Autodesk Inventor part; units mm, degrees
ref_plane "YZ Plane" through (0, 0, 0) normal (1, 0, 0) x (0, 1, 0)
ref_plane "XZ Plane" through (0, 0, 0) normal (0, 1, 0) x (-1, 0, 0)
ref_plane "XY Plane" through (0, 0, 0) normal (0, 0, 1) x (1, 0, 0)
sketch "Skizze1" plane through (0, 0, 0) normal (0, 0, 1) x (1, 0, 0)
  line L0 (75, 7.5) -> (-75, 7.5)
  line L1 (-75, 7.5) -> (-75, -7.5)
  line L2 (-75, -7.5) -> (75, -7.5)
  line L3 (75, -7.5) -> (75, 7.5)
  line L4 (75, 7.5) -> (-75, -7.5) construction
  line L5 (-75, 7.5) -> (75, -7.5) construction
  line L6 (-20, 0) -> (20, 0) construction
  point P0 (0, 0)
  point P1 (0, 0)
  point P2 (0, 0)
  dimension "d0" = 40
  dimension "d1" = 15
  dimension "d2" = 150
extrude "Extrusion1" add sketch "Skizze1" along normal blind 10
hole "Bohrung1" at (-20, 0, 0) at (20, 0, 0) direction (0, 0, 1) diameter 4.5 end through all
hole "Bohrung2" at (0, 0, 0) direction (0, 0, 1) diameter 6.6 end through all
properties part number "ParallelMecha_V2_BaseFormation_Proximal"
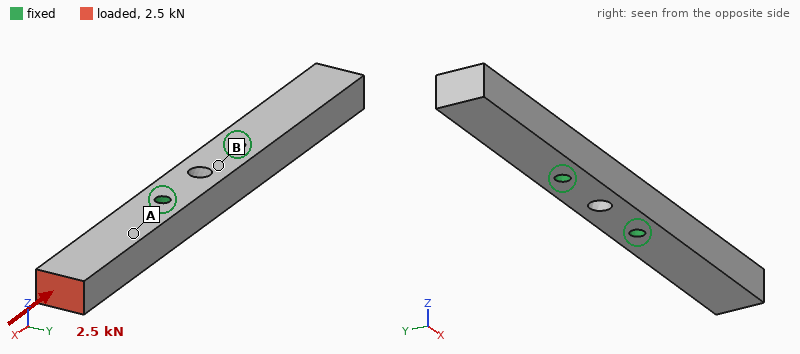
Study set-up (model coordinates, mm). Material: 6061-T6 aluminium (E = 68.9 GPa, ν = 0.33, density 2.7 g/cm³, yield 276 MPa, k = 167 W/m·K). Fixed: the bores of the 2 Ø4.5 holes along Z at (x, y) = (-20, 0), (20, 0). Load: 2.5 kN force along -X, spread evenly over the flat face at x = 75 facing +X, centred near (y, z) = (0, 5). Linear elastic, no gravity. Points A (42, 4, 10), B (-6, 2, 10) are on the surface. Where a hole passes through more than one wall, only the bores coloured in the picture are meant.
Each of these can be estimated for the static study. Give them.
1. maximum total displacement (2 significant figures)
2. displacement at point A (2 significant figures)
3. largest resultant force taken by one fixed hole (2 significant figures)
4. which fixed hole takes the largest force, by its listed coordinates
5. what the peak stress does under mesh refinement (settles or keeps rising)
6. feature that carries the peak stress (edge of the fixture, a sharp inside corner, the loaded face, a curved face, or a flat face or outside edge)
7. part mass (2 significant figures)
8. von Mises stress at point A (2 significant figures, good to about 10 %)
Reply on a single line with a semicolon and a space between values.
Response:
14 µm; 5.7 µm; 2.4 kN; (20, 0); keeps rising; edge of the fixture; 59 g; 17 MPa
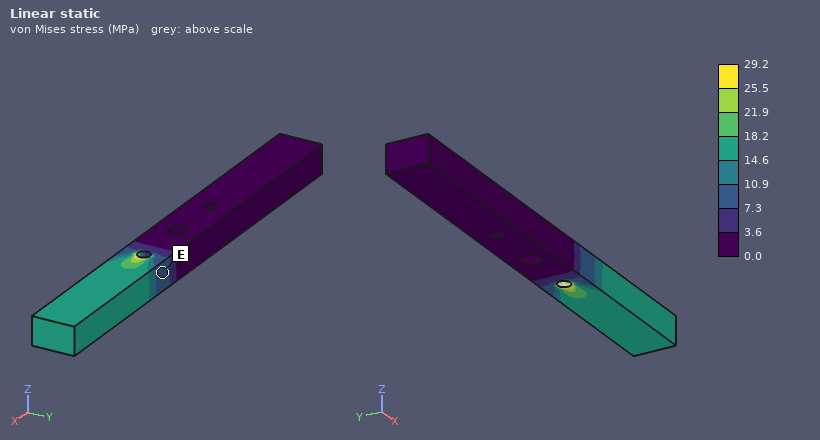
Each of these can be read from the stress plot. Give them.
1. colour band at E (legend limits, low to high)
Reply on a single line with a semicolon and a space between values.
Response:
7.3 to 10.9 MPa
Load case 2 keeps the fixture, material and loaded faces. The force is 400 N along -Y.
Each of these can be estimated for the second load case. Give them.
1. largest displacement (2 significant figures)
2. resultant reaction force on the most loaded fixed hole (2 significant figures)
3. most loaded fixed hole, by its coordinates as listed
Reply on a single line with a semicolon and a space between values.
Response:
0.16 mm; 650 N; (20, 0)
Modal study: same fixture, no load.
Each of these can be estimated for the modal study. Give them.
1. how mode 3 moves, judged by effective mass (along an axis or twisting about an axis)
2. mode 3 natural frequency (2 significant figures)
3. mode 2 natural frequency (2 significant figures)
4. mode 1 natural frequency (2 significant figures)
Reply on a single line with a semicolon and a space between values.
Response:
along Y; 3200 Hz; 2600 Hz; 2600 Hz
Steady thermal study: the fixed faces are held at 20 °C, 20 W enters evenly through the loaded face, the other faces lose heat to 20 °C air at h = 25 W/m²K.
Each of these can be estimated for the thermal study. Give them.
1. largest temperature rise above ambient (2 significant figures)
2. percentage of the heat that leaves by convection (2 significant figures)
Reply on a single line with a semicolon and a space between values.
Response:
42 K; 7.1 %
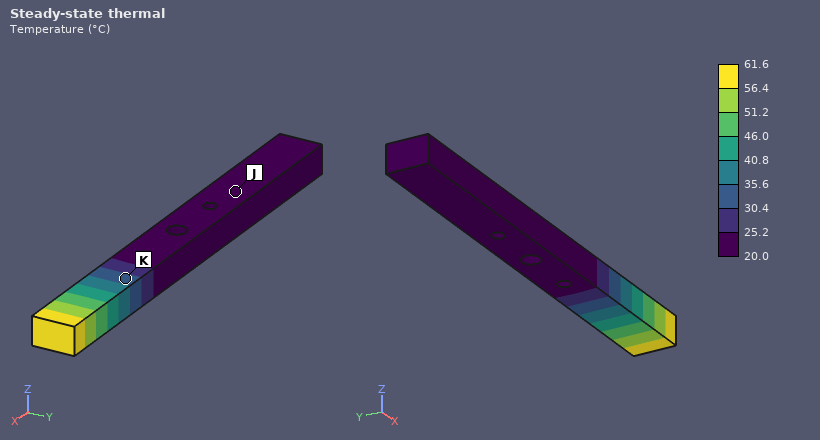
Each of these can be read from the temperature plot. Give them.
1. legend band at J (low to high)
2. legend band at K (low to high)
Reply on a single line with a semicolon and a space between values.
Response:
20.0 to 25.2 °C; 30.4 to 35.6 °C
